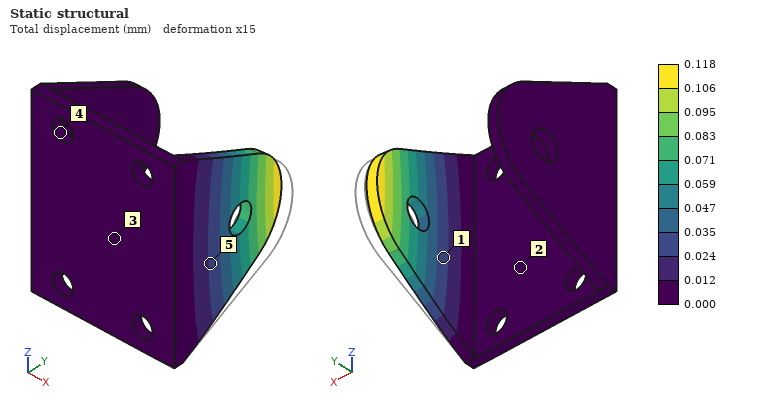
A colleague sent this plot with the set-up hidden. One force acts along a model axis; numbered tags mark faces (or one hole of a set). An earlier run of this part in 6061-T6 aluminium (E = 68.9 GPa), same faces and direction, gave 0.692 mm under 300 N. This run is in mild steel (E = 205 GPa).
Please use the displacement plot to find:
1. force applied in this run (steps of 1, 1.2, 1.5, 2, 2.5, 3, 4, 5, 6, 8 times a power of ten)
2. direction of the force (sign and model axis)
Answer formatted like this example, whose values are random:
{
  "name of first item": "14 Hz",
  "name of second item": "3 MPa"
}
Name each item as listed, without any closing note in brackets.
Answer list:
{
  "force applied in this run": "150 N",
  "direction of the force": "-X"
}
